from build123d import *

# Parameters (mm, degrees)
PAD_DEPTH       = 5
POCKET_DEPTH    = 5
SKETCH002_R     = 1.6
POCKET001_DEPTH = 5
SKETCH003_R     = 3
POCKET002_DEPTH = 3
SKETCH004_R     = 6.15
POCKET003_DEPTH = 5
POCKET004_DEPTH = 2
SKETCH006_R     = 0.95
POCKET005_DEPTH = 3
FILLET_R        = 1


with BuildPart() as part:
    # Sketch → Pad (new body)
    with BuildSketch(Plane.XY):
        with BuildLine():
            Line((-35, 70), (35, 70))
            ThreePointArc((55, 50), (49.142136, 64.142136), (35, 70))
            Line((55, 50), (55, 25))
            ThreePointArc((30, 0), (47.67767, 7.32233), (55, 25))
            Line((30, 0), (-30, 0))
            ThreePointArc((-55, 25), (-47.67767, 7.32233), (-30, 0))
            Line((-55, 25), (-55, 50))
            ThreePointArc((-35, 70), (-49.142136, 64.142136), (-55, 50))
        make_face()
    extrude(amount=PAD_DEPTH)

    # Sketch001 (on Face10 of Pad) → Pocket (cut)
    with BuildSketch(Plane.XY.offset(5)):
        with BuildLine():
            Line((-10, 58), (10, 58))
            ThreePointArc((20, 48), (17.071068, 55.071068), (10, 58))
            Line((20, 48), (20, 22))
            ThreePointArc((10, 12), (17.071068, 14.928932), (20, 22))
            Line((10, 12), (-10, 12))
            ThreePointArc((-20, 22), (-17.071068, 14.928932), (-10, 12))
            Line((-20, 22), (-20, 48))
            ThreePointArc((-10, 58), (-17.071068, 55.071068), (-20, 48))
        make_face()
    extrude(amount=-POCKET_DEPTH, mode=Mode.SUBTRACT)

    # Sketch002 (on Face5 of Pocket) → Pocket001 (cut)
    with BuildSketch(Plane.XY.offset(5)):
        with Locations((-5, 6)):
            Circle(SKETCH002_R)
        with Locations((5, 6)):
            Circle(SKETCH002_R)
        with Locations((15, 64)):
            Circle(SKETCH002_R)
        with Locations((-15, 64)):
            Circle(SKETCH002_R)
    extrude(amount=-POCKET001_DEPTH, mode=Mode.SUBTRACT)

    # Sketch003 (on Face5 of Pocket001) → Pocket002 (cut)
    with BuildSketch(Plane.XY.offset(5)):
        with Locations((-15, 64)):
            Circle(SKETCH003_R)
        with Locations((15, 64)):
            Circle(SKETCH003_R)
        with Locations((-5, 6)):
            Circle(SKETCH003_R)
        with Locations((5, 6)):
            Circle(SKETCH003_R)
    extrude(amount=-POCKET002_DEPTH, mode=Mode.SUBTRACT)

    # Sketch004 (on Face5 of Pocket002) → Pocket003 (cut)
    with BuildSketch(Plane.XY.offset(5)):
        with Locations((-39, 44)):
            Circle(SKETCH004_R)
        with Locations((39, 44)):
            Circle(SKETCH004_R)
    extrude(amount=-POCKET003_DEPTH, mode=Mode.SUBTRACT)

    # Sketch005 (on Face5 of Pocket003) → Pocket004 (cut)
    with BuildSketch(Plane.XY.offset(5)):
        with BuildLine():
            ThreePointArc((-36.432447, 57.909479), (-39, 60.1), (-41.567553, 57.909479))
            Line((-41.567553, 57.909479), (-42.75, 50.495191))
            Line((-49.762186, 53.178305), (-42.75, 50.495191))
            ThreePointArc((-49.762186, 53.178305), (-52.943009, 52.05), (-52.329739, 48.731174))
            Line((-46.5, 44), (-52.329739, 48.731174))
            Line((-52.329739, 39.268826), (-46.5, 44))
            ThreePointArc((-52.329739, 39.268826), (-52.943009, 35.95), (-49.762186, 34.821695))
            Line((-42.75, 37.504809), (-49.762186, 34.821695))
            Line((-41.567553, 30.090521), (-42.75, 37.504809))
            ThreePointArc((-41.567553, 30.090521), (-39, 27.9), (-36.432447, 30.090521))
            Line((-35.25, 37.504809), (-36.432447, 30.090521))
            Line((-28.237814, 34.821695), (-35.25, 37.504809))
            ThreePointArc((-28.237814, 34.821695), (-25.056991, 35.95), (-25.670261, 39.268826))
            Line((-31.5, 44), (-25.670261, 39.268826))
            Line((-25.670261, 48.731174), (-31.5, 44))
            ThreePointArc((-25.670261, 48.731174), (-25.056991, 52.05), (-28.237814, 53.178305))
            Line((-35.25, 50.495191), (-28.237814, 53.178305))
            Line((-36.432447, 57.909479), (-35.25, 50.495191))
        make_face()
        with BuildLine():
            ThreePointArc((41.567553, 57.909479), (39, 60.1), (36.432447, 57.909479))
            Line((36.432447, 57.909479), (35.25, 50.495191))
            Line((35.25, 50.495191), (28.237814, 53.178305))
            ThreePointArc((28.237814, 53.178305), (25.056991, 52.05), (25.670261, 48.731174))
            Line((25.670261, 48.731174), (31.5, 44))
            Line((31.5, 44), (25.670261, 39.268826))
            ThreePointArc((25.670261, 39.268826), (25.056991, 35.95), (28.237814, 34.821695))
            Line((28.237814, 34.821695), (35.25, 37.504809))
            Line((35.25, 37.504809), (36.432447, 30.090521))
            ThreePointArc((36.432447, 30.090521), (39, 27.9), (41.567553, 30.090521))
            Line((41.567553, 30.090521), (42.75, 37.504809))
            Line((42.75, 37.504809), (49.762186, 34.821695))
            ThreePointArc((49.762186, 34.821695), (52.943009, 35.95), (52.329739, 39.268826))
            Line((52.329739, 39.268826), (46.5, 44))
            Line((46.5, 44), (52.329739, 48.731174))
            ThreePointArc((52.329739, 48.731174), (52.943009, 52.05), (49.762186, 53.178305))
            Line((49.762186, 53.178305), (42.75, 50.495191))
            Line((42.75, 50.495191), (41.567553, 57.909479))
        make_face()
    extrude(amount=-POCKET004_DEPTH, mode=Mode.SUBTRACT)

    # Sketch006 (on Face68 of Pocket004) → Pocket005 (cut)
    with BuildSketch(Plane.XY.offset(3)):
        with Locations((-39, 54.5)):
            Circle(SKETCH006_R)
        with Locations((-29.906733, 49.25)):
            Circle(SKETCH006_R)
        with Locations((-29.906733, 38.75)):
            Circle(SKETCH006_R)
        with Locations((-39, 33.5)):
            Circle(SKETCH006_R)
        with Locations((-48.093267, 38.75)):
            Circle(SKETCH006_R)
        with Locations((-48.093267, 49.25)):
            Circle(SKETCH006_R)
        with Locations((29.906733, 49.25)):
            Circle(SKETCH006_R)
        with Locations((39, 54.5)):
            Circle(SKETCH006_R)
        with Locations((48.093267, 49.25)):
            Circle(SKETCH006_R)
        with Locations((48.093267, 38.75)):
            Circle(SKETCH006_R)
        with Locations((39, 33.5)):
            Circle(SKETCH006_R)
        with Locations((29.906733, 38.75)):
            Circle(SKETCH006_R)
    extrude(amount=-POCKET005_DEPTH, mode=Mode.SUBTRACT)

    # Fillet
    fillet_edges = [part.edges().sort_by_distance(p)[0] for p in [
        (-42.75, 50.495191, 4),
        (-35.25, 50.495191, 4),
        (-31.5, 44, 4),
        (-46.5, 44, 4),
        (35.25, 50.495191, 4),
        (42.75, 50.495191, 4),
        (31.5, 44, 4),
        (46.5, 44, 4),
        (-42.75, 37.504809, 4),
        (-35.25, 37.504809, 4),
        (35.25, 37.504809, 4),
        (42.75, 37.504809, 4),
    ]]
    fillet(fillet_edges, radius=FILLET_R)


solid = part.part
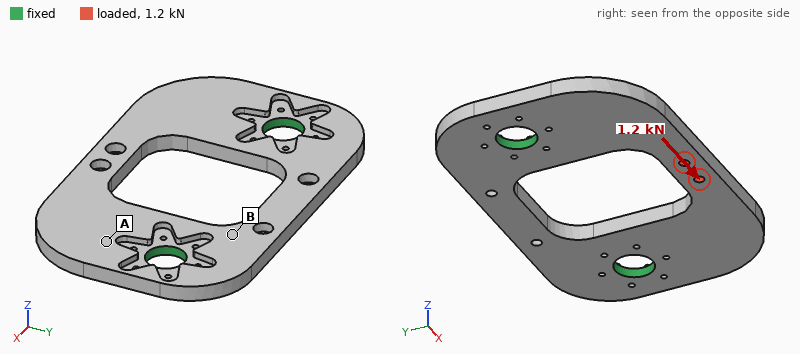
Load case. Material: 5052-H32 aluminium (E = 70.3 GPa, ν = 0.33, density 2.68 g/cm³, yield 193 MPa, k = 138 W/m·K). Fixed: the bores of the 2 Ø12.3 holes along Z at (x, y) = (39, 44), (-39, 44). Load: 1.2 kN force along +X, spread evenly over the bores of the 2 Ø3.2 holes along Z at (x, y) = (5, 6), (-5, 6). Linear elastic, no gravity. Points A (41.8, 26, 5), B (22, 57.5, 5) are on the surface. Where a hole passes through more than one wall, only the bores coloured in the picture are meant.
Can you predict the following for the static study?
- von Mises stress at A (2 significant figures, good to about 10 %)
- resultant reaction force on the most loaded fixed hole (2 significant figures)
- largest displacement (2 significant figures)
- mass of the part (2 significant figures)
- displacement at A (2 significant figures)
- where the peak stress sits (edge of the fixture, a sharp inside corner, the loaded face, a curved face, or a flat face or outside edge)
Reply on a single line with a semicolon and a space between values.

9.1 MPa; 670 N; 31 µm; 65 g; 11 µm; the loaded face
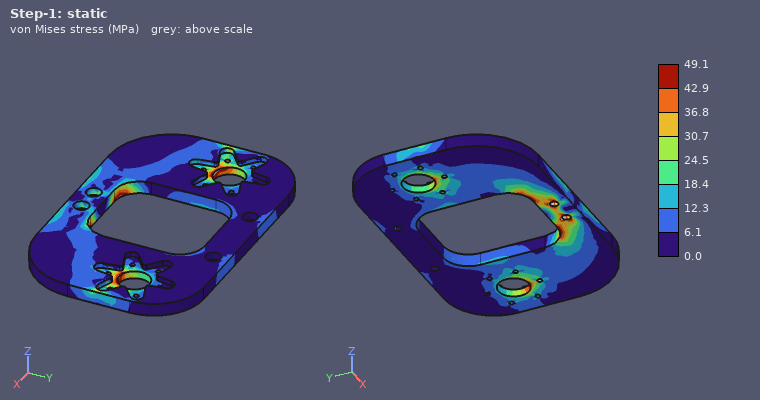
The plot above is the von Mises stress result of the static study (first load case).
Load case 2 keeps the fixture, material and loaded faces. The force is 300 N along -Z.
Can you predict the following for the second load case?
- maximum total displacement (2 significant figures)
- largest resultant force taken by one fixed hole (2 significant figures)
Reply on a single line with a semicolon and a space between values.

0.31 mm; 160 N
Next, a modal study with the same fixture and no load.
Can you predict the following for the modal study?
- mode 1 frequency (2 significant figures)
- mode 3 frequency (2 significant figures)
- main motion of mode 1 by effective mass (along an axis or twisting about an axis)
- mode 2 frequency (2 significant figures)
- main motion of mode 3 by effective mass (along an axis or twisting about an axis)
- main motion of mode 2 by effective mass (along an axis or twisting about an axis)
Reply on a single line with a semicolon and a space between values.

1600 Hz; 3300 Hz; along Z; 2700 Hz; along Z; twisting about Y
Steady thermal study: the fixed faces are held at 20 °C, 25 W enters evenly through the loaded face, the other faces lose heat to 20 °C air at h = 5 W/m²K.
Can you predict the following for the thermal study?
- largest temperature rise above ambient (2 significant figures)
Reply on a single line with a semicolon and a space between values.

59 K
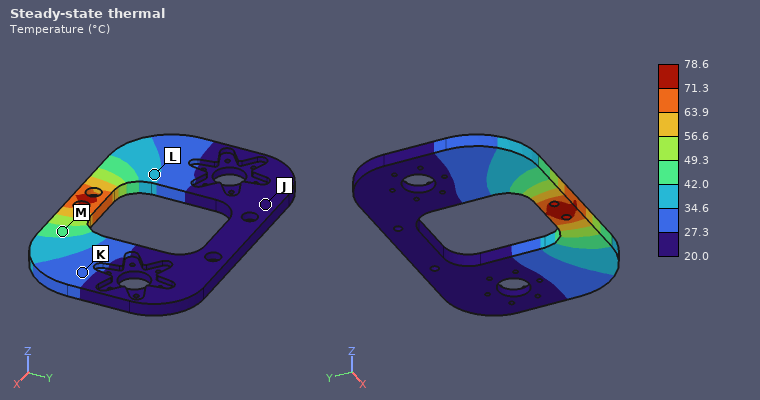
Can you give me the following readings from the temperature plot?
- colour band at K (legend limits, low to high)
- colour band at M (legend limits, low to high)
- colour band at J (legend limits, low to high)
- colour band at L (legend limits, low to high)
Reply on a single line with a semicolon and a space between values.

27.3 to 34.6 °C; 42.0 to 49.3 °C; 20.0 to 27.3 °C; 34.6 to 42.0 °C
